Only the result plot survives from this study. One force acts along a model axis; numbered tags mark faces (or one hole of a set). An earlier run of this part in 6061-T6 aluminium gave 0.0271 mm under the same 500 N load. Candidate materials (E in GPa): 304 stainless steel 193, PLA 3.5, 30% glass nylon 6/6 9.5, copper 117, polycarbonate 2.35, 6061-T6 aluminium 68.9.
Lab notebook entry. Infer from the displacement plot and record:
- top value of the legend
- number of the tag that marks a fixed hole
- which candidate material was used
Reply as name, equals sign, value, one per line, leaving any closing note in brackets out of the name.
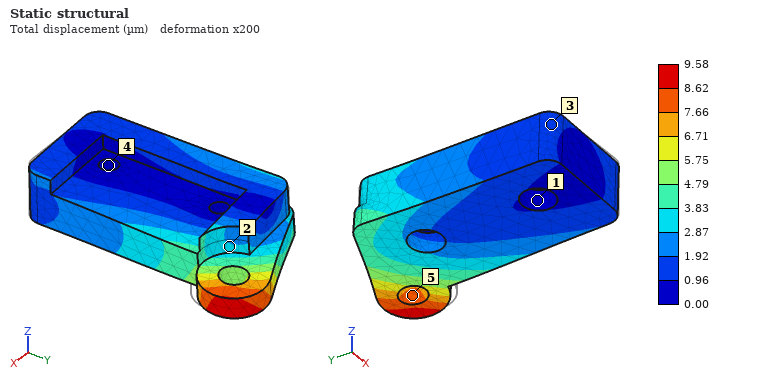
top value of the legend = 9.58 µm
number of the tag that marks a fixed hole = 4
which candidate material was used = 304 stainless steel
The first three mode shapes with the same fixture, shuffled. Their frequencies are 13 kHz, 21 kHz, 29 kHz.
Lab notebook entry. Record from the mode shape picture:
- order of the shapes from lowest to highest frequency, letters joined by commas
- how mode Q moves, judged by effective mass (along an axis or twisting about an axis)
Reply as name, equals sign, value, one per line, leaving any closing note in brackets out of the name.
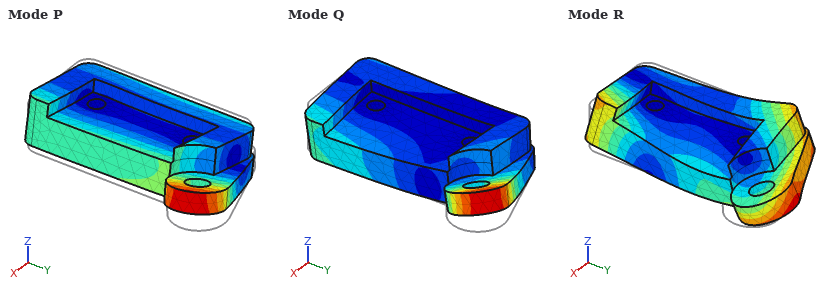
order of the shapes from lowest to highest frequency, letters joined by commas = P, Q, R
how mode Q moves, judged by effective mass = twisting about X
